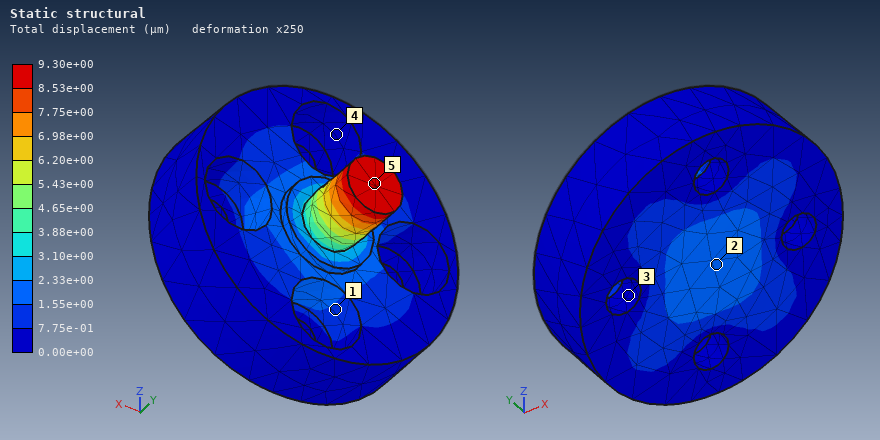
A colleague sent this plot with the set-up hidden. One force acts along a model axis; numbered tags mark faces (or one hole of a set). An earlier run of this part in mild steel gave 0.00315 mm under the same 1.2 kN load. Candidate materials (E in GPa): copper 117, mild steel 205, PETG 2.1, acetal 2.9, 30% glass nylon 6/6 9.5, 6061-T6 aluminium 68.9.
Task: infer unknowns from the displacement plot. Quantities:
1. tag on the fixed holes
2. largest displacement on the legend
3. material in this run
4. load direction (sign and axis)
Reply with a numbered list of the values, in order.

1. 3
2. 9.30e+00 µm
3. 6061-T6 aluminium
4. -Y
